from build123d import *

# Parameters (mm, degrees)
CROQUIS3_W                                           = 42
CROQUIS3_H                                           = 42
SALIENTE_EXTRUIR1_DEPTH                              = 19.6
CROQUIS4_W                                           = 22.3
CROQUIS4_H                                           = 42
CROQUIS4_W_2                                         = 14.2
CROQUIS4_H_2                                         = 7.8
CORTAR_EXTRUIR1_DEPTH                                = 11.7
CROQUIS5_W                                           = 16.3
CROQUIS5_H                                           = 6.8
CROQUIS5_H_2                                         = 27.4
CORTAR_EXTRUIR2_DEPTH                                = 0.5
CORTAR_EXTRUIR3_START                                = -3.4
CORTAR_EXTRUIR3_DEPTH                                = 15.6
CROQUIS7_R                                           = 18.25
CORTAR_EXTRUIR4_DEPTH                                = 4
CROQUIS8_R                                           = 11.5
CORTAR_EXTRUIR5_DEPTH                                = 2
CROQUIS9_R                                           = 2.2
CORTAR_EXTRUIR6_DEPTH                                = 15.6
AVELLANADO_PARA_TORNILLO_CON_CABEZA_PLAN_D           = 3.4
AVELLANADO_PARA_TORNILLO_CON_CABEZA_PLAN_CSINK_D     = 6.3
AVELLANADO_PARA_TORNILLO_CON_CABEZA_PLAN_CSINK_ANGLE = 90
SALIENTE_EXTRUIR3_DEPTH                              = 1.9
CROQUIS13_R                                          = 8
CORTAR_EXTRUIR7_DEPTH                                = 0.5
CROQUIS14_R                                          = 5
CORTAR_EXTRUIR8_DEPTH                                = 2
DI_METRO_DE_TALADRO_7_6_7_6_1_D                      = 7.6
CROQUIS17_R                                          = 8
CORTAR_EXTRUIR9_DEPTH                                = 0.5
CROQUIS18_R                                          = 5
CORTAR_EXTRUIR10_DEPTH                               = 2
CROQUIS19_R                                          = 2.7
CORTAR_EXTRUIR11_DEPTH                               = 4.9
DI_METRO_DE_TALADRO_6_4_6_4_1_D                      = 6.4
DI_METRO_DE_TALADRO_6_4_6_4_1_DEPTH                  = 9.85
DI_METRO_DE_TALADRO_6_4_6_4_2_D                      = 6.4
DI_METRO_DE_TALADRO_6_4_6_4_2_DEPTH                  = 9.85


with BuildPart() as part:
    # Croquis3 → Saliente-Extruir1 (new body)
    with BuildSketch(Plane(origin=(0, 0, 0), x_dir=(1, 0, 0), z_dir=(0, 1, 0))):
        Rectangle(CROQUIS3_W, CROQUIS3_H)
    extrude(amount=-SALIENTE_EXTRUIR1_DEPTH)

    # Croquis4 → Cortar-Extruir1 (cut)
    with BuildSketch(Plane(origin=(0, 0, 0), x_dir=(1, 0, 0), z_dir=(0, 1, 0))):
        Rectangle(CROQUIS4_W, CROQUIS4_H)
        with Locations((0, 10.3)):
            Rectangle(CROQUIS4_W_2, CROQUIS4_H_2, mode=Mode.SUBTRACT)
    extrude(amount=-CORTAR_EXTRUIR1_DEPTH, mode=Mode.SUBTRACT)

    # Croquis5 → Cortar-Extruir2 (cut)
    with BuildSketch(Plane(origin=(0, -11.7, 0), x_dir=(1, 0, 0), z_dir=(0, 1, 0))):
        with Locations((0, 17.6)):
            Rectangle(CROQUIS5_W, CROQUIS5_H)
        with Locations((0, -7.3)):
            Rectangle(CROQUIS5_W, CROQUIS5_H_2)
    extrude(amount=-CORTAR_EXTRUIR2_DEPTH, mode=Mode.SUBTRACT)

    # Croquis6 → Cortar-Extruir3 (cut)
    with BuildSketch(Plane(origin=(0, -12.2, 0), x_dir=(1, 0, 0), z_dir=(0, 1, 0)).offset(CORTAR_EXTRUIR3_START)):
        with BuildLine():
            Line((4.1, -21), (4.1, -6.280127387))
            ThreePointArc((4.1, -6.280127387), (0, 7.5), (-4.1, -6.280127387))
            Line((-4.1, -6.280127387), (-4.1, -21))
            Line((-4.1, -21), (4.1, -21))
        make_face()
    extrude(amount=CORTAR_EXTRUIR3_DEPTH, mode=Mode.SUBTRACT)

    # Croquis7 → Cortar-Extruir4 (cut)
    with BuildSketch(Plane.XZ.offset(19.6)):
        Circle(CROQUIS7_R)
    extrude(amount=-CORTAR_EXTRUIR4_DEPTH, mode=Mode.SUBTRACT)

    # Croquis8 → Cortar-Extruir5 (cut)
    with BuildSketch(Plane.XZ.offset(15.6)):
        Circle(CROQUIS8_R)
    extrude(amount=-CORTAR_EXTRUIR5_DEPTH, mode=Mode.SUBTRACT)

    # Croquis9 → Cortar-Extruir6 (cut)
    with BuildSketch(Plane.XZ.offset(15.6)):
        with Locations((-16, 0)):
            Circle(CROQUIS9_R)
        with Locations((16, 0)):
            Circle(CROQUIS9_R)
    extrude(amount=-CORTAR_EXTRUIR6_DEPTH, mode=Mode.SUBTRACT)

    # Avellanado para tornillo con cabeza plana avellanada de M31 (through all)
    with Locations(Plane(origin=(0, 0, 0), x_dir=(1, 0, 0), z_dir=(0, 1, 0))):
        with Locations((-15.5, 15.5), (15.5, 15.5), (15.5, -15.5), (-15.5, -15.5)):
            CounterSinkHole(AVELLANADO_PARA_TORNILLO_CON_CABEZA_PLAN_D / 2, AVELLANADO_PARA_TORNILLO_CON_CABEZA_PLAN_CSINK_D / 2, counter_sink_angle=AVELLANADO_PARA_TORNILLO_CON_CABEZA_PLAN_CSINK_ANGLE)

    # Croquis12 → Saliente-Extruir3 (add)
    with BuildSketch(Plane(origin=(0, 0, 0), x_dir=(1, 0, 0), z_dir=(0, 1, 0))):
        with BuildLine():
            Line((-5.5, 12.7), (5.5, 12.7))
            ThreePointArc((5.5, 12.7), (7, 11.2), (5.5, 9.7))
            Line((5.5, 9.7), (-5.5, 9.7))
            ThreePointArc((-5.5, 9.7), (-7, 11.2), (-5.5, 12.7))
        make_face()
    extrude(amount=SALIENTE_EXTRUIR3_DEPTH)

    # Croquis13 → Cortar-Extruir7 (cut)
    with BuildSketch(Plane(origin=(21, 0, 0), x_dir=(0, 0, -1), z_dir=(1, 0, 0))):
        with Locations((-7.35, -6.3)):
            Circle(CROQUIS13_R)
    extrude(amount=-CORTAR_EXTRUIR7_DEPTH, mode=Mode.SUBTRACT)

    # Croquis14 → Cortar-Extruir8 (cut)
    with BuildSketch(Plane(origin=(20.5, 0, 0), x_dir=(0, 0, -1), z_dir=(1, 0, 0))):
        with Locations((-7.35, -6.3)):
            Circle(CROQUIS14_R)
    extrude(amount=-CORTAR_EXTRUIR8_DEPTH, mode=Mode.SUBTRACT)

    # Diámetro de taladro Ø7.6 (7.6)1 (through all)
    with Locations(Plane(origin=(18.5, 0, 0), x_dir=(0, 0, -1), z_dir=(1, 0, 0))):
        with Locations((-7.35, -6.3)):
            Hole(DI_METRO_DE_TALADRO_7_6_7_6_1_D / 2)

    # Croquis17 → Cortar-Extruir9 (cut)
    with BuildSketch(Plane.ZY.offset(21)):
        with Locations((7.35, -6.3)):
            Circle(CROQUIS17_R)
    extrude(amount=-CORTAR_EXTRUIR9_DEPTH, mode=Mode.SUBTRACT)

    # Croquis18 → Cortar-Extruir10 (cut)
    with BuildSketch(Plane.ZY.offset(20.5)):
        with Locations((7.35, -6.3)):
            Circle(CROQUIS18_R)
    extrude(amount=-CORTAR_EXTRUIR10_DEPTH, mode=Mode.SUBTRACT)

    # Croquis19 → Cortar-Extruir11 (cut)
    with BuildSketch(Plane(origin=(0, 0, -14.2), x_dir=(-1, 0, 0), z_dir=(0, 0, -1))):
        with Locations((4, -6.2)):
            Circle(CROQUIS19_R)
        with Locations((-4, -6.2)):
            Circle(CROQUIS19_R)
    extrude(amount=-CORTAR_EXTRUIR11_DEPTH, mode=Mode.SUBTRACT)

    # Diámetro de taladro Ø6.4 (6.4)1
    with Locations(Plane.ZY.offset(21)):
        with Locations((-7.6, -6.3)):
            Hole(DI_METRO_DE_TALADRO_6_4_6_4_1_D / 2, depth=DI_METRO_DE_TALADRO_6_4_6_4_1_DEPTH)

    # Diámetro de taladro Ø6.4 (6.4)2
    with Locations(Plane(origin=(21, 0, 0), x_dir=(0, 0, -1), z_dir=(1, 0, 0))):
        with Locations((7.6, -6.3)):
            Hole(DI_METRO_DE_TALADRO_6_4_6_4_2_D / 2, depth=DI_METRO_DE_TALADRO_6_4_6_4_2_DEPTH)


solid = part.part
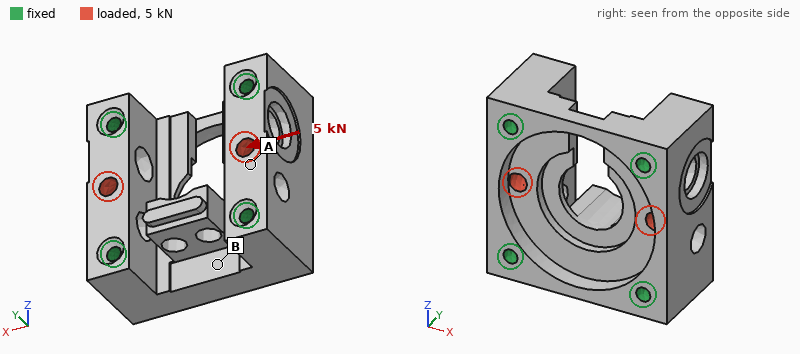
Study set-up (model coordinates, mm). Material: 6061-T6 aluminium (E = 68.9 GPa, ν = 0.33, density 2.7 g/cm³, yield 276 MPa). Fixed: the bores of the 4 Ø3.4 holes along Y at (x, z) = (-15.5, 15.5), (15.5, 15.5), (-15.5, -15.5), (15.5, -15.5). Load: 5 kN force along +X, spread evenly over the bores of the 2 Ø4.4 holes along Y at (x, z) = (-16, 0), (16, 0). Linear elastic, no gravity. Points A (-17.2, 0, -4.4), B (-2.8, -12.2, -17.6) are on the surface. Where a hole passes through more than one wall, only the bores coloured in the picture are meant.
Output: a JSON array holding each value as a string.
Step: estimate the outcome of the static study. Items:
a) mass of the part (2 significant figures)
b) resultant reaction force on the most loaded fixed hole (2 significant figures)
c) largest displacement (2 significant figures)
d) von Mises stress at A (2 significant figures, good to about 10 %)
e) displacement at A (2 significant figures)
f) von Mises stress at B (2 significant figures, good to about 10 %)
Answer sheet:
["43 g", "1.4 kN", "17 µm", "30 MPa", "13 µm", "11 MPa"]
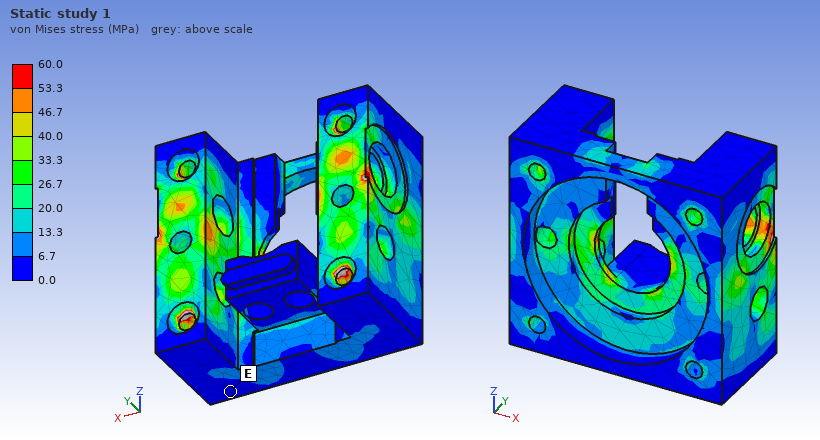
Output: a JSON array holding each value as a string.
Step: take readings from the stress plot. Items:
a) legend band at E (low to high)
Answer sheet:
["0.0 to 6.7 MPa"]
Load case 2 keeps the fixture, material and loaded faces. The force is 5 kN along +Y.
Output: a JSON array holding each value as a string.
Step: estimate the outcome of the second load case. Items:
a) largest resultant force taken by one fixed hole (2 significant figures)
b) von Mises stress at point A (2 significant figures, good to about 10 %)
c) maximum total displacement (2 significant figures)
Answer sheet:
["1.4 kN", "12 MPa", "12 µm"]
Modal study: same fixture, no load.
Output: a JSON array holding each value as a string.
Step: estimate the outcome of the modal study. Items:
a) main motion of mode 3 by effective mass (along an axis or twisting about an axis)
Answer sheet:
["along Y"]
